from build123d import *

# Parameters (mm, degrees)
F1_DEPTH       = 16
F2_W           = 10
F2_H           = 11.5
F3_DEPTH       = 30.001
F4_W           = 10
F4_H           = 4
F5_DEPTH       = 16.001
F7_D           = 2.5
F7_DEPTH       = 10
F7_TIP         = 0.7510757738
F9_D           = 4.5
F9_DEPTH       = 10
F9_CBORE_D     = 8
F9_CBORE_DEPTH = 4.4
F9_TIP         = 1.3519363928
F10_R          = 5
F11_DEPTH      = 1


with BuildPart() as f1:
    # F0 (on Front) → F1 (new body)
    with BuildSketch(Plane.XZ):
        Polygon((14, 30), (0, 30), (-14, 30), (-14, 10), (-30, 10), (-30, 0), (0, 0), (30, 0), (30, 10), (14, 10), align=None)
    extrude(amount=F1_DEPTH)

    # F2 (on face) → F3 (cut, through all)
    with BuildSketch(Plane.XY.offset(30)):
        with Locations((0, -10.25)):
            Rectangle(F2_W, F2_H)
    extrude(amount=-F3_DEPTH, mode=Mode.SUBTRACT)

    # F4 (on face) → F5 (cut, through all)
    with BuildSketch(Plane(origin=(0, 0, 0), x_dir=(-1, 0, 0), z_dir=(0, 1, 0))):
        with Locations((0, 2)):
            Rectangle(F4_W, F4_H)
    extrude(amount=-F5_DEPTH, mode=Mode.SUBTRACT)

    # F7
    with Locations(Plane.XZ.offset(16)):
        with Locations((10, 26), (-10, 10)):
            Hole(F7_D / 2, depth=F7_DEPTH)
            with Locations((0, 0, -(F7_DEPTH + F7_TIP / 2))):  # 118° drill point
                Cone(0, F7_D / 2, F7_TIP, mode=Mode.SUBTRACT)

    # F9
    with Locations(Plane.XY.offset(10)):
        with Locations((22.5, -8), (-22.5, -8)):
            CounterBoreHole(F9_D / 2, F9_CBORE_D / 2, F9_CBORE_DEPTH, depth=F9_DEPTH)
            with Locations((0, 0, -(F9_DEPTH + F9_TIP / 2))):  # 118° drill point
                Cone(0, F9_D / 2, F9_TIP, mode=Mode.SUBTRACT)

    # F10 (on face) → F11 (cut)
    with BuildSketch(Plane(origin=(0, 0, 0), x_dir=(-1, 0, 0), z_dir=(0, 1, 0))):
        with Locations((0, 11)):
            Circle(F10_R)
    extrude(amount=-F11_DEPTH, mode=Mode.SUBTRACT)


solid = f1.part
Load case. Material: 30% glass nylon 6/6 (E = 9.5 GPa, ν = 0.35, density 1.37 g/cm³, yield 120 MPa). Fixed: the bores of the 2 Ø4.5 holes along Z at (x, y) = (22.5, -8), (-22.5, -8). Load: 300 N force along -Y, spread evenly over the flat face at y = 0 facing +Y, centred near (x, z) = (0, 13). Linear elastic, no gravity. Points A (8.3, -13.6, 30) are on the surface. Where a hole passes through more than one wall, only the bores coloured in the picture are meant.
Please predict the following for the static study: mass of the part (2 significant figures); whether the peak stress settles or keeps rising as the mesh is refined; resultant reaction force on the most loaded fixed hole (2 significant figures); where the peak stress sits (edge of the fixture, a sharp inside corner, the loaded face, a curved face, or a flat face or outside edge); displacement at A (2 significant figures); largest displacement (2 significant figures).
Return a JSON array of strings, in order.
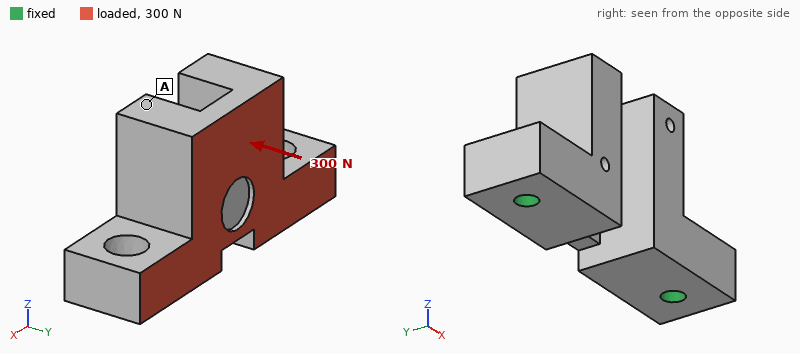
["19 g", "keeps rising", "160 N", "edge of the fixture", "76 µm", "82 µm"]
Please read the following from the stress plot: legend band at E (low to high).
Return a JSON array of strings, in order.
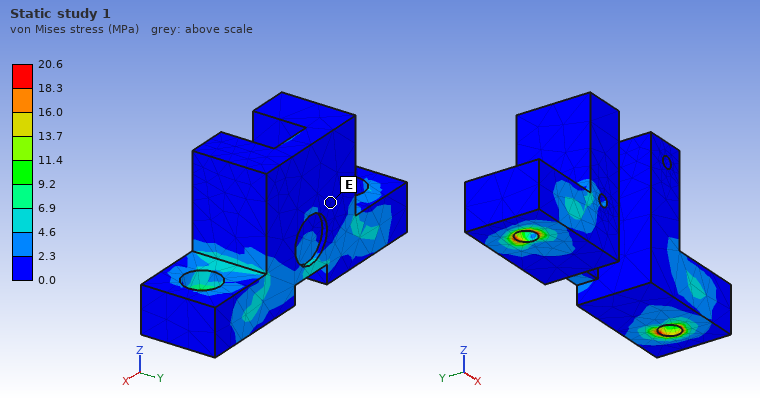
["0.0 to 2.3 MPa"]
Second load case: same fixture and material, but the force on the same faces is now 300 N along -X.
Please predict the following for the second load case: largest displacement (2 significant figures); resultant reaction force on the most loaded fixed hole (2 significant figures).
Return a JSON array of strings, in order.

["11 µm", "170 N"]
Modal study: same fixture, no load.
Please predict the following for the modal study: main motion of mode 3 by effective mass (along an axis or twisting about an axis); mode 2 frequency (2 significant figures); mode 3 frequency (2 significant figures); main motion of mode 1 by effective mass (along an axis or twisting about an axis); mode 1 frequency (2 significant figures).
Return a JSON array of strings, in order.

["along Z", "5400 Hz", "6200 Hz", "along Y", "2800 Hz"]
